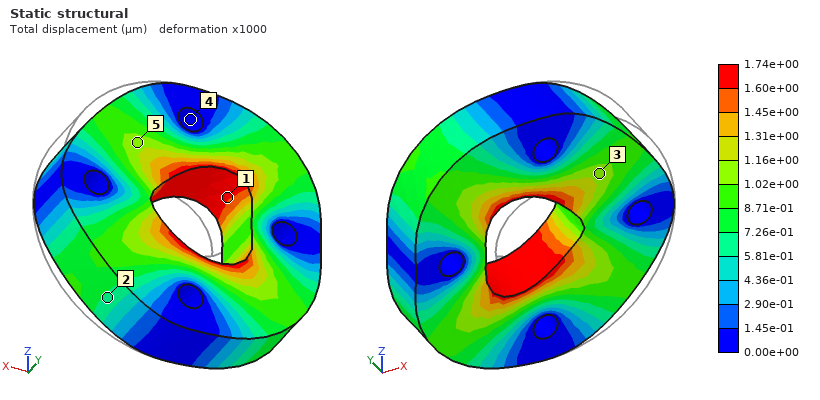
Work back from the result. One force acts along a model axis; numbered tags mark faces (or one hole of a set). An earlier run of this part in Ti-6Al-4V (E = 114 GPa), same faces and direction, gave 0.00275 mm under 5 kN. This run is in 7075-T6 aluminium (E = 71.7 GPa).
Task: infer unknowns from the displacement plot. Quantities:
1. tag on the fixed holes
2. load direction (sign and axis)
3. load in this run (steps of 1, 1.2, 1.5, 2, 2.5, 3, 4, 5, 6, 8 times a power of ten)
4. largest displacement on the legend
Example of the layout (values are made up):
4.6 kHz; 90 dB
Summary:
4; -X; 2 kN; 1.74e+00 µm
